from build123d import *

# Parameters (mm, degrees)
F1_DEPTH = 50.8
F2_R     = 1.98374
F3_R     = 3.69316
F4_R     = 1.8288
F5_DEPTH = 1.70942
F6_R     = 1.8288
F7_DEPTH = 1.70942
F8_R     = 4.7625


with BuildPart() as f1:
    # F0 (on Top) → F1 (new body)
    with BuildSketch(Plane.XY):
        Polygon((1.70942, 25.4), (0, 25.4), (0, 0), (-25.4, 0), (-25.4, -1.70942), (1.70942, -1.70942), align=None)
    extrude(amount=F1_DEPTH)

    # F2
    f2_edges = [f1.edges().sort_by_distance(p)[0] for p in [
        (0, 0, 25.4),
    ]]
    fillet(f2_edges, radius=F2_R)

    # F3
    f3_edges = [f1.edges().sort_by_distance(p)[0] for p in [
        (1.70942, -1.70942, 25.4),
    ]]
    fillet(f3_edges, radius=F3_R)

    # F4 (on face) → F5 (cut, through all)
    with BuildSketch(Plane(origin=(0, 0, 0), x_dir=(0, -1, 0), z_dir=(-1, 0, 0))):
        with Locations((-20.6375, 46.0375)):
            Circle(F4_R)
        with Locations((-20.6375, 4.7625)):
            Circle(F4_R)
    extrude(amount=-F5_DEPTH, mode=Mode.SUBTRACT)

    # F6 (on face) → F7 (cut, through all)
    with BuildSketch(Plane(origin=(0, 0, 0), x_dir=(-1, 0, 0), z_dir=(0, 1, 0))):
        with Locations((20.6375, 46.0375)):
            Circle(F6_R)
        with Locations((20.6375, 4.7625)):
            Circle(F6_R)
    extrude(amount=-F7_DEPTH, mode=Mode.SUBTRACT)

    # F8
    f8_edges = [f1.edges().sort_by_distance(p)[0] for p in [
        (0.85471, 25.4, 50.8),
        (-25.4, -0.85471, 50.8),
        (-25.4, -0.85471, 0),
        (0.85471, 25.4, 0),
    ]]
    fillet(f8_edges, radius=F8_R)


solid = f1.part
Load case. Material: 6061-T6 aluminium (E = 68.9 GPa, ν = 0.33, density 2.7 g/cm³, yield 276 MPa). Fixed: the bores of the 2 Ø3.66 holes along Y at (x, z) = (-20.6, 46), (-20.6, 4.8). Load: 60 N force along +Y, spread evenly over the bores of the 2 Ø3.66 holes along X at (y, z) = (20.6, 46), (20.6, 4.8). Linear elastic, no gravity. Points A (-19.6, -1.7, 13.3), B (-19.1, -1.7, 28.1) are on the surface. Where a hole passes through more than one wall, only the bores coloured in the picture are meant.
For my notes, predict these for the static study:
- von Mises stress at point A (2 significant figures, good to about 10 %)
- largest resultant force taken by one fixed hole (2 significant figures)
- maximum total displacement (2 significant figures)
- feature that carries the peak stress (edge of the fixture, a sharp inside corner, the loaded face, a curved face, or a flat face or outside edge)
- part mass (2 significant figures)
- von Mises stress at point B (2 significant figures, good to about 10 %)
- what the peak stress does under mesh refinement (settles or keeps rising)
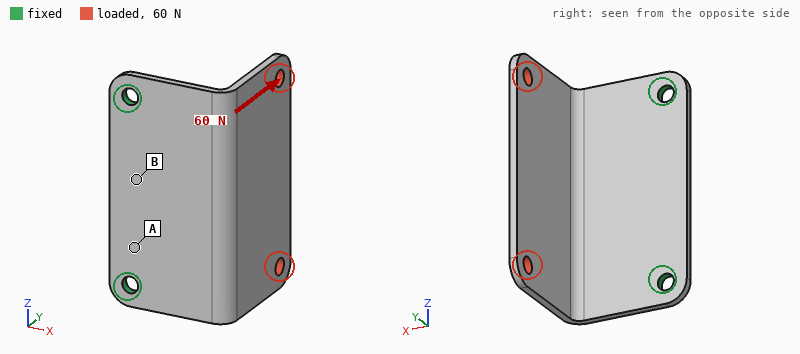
31 MPa
30 N
0.34 mm
edge of the fixture
12 g
12 MPa
keeps rising
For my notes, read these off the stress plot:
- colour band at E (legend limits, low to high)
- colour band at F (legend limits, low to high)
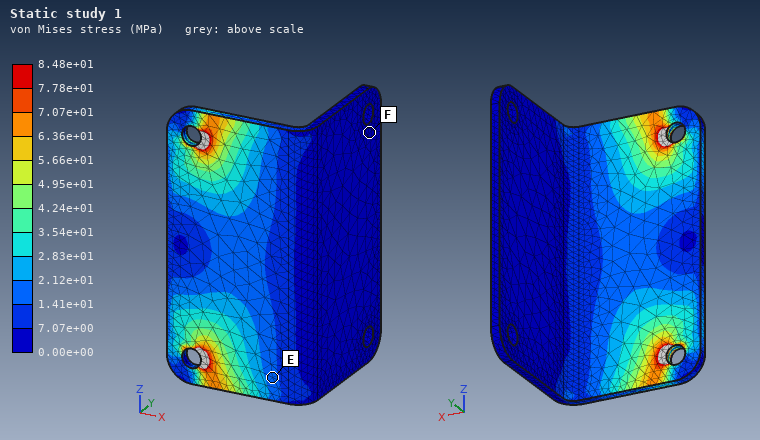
1.41e+01 to 2.12e+01 MPa
0.00e+00 to 7.07e+00 MPa
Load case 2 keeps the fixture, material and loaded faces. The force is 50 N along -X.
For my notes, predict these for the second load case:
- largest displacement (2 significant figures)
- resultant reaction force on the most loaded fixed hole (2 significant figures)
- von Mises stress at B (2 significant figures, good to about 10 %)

0.61 mm
27 N
15 MPa
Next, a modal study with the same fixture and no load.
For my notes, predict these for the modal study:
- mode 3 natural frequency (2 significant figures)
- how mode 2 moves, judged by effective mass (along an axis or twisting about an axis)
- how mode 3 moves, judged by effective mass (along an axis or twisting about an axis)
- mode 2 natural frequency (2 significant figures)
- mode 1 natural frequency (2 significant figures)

2200 Hz
along Z
along Y
1600 Hz
790 Hz
